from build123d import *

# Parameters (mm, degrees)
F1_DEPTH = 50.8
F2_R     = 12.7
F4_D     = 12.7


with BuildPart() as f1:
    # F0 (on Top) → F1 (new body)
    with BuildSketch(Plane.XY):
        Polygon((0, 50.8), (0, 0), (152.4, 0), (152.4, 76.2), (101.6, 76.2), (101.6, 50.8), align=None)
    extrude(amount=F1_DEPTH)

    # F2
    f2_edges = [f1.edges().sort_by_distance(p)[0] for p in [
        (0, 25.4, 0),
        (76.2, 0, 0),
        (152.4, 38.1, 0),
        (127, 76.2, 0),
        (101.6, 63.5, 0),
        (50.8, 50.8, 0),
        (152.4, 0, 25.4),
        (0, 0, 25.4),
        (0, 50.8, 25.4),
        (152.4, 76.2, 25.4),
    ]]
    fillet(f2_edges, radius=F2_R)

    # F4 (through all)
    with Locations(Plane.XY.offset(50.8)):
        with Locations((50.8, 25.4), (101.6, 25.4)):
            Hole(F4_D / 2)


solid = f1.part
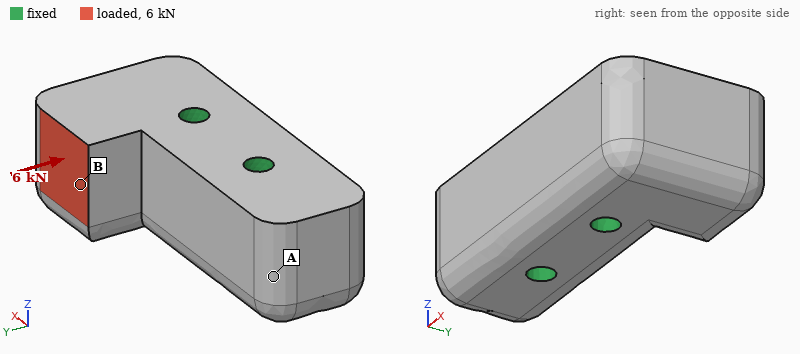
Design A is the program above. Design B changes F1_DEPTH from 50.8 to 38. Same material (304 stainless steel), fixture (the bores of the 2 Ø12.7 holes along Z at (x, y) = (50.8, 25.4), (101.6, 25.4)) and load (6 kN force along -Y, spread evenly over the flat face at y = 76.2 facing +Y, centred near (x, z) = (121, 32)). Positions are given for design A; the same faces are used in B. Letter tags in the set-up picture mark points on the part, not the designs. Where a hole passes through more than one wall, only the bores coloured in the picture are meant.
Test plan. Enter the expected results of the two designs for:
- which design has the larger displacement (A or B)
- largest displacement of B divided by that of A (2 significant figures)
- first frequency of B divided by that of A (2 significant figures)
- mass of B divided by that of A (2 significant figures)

B
1.5
1.00
0.74
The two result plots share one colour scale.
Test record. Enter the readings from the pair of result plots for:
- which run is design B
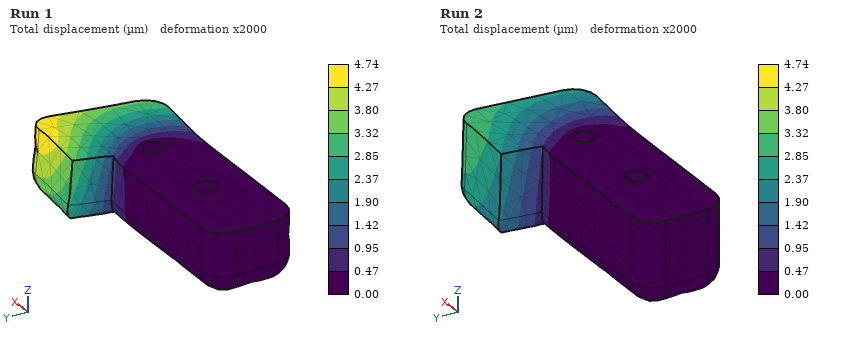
Run 1
